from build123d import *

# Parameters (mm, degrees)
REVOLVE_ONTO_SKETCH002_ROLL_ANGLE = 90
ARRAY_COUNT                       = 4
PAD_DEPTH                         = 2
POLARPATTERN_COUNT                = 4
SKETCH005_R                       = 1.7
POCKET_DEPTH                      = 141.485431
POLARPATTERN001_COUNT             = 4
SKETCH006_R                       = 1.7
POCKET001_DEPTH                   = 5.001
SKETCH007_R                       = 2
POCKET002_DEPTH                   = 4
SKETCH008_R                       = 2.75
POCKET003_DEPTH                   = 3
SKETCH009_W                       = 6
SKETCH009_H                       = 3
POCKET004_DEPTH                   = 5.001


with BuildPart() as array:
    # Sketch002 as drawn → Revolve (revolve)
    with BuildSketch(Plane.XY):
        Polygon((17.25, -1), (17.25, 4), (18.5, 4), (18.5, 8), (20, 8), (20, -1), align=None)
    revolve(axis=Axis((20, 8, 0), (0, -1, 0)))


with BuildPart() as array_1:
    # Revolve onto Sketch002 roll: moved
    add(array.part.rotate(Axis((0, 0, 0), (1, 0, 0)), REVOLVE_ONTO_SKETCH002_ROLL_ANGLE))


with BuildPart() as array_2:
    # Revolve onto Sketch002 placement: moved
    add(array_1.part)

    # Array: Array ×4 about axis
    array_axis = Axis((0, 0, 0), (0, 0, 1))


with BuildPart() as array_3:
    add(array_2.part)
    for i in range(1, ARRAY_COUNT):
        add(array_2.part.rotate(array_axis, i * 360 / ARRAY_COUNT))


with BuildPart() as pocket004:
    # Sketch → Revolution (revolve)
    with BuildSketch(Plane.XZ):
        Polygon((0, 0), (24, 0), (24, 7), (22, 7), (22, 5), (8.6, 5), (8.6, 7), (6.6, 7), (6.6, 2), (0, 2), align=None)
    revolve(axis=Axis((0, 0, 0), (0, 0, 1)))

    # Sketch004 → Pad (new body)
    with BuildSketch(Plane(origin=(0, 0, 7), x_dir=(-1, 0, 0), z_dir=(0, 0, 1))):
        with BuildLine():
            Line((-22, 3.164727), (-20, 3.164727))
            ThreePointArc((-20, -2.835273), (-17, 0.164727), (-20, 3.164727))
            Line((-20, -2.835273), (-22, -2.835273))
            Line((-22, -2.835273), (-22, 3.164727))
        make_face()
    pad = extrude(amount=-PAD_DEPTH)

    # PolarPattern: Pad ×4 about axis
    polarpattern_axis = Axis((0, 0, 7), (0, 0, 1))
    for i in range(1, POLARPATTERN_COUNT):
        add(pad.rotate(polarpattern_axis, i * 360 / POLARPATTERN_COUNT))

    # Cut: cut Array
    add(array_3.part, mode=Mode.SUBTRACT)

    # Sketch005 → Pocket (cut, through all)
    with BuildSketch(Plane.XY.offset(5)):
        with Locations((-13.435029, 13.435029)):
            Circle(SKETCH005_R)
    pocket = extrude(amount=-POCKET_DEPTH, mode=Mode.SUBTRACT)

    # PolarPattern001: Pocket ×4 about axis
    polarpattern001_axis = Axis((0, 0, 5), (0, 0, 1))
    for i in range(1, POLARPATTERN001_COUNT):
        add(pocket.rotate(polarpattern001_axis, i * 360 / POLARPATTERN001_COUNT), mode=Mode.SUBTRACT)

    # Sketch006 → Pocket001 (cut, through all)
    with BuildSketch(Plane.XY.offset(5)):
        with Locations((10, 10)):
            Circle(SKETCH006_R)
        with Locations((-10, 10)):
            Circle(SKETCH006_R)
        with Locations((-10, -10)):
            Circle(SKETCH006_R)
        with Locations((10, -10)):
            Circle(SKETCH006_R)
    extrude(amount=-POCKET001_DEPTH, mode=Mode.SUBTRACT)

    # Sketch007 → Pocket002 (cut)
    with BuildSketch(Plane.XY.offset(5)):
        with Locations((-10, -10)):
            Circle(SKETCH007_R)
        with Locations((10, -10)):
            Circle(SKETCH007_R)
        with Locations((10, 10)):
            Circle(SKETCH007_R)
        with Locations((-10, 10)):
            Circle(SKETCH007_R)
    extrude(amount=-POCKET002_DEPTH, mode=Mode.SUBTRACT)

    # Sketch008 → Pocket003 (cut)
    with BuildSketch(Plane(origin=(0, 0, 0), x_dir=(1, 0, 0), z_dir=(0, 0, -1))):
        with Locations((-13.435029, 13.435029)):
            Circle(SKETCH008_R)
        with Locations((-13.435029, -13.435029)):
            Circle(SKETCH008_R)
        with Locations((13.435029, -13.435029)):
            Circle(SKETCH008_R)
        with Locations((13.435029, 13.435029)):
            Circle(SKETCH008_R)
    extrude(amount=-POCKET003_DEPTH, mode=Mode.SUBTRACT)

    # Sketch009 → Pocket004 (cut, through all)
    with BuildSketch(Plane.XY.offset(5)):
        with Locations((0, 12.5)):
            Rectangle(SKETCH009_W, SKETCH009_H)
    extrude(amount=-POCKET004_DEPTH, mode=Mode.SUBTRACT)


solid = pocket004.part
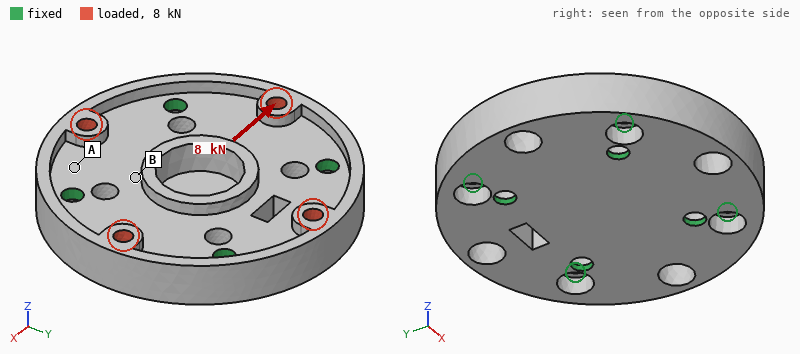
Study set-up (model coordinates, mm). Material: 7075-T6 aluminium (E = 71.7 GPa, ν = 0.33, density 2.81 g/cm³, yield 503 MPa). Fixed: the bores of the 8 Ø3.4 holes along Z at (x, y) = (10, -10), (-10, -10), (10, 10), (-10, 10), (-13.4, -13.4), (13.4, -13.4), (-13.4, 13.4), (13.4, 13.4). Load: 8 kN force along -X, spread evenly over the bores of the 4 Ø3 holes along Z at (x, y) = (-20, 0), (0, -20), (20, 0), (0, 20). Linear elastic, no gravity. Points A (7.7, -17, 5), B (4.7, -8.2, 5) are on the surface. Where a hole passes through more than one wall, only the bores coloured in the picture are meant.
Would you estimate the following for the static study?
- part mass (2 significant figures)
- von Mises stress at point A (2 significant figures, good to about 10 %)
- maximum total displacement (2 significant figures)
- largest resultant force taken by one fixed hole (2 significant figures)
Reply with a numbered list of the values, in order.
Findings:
1. 24 g
2. 39 MPa
3. 43 µm
4. 1.5 kN
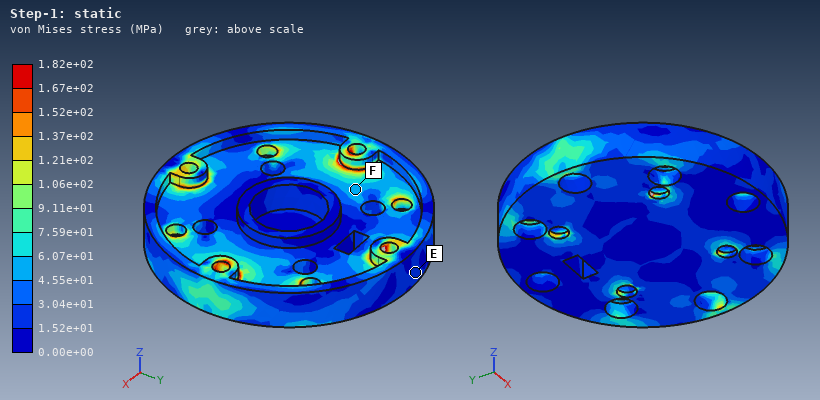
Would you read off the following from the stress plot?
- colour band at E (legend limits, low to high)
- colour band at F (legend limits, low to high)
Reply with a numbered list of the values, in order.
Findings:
1. 1.52e+01 to 3.04e+01 MPa
2. 4.55e+01 to 6.07e+01 MPa
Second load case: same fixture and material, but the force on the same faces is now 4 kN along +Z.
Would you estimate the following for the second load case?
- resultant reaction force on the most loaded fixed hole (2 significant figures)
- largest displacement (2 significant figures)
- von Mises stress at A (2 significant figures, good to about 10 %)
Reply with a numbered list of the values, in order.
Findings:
1. 620 N
2. 36 µm
3. 27 MPa
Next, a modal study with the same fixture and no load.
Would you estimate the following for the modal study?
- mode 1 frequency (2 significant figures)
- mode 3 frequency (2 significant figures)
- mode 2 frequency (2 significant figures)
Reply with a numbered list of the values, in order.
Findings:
1. 19 kHz
2. 21 kHz
3. 21 kHz
